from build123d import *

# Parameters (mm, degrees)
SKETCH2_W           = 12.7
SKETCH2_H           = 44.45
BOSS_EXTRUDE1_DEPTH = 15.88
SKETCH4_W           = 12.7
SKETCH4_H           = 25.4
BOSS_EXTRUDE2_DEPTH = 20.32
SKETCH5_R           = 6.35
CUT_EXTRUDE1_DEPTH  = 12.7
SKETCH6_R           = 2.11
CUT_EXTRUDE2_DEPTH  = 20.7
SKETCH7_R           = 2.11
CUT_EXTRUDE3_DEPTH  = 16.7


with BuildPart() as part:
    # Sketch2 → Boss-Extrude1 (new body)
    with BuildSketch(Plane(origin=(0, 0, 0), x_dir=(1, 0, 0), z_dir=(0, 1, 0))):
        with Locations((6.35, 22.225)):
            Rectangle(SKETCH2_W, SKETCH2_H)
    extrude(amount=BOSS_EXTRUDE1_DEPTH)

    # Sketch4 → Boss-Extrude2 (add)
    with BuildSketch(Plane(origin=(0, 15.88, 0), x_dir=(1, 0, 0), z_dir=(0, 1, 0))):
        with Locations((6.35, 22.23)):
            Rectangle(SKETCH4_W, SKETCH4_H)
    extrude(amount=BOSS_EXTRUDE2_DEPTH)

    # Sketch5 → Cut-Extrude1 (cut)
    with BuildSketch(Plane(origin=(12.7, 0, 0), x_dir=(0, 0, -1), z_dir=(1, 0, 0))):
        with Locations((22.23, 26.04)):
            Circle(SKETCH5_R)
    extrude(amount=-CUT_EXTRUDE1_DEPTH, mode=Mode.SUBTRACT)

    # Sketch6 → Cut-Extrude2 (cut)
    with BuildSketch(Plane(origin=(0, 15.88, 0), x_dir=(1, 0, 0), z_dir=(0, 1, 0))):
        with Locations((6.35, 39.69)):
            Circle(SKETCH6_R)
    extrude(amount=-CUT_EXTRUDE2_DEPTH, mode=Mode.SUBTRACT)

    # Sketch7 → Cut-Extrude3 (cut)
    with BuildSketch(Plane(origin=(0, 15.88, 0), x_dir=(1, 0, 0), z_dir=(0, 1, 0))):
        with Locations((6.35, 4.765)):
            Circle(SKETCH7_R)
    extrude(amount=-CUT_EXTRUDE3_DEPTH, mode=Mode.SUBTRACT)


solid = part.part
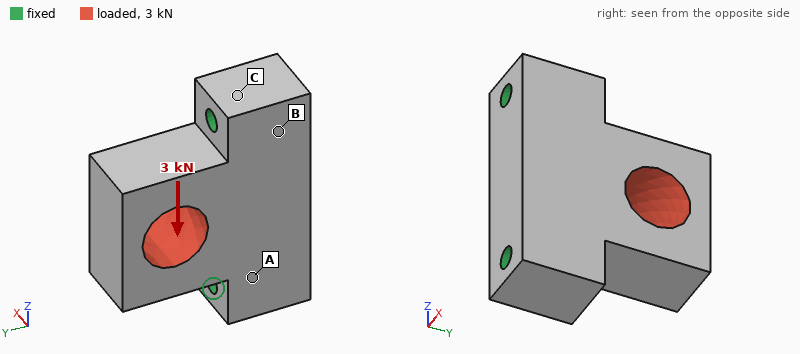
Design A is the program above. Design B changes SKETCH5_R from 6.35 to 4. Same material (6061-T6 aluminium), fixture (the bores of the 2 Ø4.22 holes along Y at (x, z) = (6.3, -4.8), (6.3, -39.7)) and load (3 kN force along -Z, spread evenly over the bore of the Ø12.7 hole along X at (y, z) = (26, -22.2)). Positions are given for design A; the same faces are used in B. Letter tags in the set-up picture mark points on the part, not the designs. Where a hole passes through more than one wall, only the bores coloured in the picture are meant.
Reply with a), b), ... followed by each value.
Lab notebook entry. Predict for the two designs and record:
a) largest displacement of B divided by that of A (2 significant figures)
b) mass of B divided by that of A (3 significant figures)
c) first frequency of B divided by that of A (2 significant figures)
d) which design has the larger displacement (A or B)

a) 0.63
b) 1.07
c) 0.95
d) A
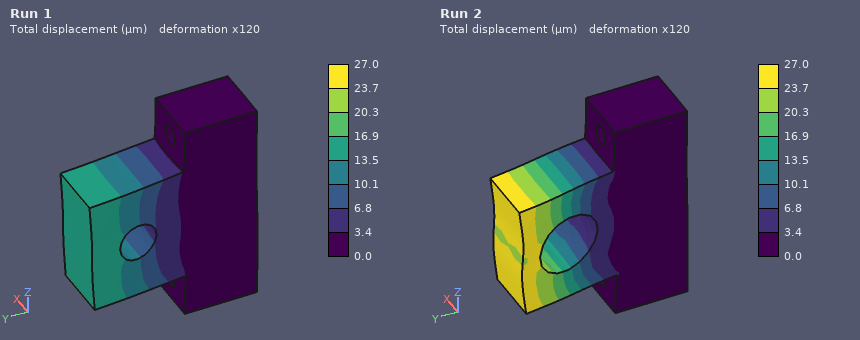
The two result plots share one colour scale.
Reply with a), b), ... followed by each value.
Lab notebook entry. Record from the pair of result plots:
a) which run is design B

a) Run 1
